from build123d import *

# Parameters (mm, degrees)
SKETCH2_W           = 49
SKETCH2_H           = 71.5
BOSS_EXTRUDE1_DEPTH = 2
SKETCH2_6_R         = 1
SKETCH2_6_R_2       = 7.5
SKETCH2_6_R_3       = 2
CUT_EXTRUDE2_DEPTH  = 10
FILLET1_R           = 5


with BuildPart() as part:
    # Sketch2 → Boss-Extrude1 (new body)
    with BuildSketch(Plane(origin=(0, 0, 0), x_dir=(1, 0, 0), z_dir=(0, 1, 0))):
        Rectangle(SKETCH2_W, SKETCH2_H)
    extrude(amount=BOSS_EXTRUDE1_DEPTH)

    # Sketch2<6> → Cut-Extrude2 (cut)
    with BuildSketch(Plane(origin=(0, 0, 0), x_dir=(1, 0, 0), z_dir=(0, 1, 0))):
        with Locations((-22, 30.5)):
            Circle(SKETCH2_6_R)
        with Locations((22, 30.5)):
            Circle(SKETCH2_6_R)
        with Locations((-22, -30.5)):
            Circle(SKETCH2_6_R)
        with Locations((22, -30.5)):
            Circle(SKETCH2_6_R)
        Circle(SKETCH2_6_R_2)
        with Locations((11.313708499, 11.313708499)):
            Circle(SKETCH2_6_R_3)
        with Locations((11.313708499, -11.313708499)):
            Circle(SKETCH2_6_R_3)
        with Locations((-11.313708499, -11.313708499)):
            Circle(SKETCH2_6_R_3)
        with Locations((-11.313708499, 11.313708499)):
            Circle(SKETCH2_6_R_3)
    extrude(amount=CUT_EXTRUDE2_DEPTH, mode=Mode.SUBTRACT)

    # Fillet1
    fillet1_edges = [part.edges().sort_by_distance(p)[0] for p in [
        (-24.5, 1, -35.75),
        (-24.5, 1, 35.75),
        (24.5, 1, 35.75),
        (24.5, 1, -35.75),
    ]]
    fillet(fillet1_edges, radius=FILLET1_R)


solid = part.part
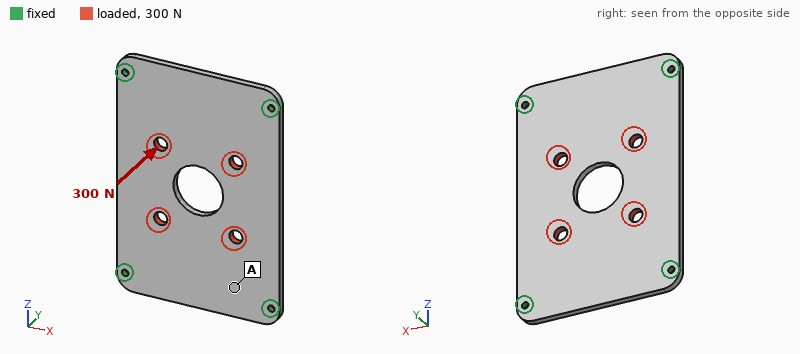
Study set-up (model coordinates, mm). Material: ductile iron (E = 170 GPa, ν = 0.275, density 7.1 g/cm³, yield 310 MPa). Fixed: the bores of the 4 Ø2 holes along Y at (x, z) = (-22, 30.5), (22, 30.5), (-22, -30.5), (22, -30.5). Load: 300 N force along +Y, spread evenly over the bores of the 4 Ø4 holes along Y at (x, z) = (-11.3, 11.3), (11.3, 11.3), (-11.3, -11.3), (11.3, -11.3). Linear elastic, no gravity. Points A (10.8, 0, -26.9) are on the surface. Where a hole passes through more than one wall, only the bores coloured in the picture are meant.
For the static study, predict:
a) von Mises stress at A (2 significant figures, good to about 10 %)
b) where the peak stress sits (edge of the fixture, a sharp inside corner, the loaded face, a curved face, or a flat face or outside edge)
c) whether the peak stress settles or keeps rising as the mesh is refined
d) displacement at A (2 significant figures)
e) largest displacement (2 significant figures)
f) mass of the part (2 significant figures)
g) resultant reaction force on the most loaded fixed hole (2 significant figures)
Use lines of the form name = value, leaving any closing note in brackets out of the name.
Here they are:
von Mises stress at A = 29 MPa
where the peak stress sits = edge of the fixture
whether the peak stress settles or keeps rising as the mesh is refined = keeps rising
displacement at A = 0.020 mm
largest displacement = 0.10 mm
mass of the part = 46 g
resultant reaction force on the most loaded fixed hole = 75 N
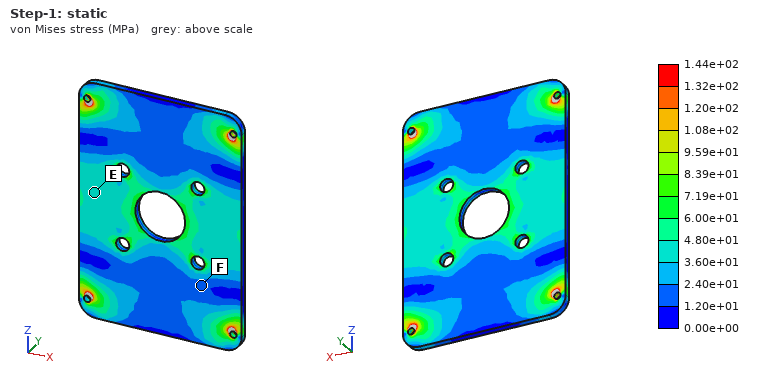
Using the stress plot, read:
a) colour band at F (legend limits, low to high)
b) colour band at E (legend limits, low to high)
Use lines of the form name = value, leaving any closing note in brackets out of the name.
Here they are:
colour band at F = 1.20e+01 to 2.40e+01 MPa
colour band at E = 3.60e+01 to 4.80e+01 MPa
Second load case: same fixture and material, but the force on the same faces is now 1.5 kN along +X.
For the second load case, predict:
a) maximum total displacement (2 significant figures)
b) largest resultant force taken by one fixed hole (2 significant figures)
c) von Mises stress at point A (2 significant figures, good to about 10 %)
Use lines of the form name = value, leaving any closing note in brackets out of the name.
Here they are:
maximum total displacement = 4.2 µm
largest resultant force taken by one fixed hole = 440 N
von Mises stress at point A = 14 MPa
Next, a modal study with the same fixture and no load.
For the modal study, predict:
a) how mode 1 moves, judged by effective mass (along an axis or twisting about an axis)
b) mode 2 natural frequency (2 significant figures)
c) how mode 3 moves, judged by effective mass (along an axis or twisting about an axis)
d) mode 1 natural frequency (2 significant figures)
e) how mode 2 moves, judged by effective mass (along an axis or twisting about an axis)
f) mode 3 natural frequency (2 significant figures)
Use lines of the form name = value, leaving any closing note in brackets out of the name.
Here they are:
how mode 1 moves, judged by effective mass = along Y
mode 2 natural frequency = 3400 Hz
how mode 3 moves, judged by effective mass = twisting about X
mode 1 natural frequency = 2000 Hz
how mode 2 moves, judged by effective mass = twisting about Z
mode 3 natural frequency = 4500 Hz
